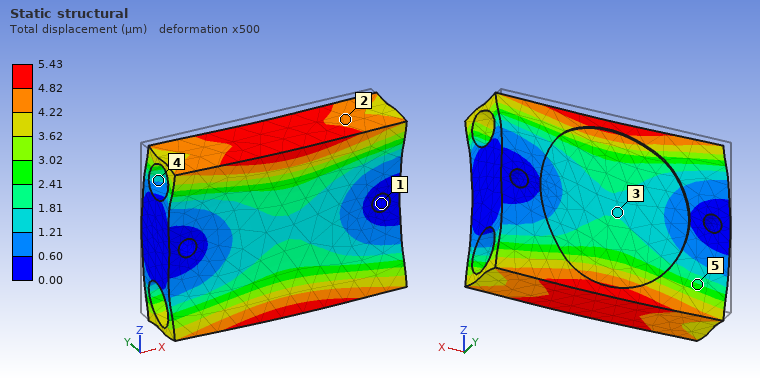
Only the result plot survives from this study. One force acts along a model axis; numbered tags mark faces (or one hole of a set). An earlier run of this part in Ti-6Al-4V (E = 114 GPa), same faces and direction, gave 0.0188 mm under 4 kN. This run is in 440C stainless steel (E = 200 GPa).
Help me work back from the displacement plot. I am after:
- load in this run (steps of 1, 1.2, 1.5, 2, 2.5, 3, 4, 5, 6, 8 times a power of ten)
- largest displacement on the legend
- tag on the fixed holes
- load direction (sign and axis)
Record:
2 kN
5.43 µm
1
-Y
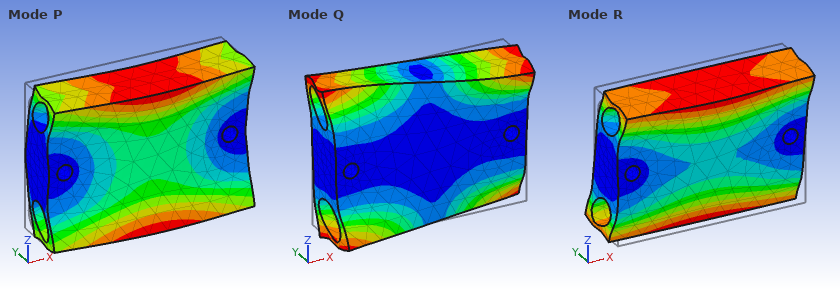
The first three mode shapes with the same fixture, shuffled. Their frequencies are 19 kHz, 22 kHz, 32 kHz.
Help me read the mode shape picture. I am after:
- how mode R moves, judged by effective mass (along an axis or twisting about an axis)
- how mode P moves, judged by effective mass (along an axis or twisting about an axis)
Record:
twisting about X
along Y
